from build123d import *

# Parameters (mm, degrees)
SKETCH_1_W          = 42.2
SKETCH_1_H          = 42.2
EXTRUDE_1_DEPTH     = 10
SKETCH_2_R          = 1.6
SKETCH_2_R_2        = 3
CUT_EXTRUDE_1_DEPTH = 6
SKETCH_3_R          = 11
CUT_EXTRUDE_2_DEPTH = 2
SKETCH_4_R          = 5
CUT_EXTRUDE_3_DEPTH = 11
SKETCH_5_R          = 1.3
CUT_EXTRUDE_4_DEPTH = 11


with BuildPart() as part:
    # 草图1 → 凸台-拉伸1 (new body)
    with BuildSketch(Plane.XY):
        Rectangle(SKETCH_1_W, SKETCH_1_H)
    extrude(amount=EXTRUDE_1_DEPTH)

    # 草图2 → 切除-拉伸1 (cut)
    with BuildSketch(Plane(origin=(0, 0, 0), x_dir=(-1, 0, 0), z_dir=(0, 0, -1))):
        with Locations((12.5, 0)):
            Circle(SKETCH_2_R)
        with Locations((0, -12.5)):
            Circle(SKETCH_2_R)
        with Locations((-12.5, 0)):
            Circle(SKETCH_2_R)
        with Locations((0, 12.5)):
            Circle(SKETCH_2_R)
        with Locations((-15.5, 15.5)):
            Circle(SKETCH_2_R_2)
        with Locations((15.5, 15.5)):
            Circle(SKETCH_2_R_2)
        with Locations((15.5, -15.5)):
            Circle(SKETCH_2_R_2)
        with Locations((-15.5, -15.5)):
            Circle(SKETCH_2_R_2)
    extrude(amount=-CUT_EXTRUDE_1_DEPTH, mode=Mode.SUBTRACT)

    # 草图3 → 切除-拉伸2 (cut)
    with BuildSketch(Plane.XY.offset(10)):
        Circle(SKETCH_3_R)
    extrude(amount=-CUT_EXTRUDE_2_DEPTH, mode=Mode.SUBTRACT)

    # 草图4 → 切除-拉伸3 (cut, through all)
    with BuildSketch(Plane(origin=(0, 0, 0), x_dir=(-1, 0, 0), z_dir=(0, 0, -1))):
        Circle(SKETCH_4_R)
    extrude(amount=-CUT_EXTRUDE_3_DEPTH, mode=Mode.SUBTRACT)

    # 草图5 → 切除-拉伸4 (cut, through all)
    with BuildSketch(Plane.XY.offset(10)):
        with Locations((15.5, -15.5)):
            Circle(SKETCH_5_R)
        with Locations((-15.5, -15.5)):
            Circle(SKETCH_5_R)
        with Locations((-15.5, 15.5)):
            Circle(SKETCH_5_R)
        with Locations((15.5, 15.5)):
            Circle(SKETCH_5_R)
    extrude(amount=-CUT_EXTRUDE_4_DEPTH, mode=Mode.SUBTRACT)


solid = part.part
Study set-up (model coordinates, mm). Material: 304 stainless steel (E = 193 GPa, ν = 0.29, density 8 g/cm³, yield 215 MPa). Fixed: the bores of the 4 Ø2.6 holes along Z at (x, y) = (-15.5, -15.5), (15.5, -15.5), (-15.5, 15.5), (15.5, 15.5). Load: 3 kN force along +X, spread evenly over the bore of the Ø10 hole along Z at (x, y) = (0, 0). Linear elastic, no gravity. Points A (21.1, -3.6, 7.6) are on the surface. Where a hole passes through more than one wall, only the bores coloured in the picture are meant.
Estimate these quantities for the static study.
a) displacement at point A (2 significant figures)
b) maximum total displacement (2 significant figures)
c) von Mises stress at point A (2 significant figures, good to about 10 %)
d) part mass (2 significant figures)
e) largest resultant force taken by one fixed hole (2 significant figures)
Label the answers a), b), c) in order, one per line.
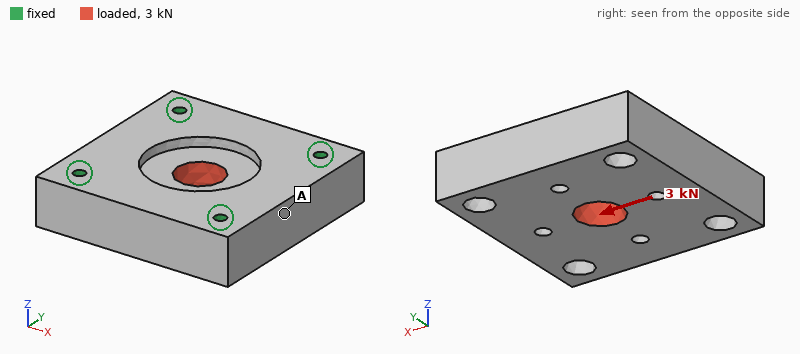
a) 1.0 µm
b) 1.8 µm
c) 7.3 MPa
d) 120 g
e) 800 N
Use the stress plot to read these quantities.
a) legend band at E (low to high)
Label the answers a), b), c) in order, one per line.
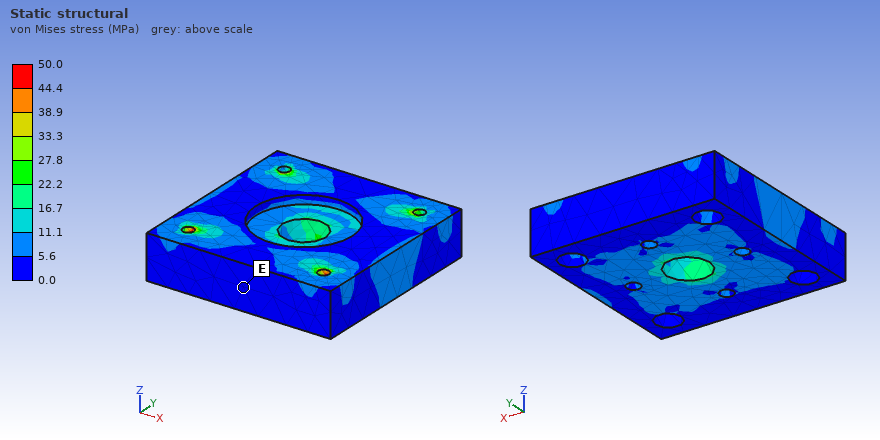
a) 0.0 to 5.6 MPa
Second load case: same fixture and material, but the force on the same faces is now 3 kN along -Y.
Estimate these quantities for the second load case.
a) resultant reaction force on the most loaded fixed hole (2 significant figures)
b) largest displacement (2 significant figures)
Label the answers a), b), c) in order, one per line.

a) 800 N
b) 1.7 µm
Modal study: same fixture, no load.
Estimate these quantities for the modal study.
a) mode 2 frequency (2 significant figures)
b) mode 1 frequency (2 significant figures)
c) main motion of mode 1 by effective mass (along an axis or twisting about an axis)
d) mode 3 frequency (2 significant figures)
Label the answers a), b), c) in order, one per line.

a) 25 kHz
b) 19 kHz
c) along Z
d) 25 kHz
